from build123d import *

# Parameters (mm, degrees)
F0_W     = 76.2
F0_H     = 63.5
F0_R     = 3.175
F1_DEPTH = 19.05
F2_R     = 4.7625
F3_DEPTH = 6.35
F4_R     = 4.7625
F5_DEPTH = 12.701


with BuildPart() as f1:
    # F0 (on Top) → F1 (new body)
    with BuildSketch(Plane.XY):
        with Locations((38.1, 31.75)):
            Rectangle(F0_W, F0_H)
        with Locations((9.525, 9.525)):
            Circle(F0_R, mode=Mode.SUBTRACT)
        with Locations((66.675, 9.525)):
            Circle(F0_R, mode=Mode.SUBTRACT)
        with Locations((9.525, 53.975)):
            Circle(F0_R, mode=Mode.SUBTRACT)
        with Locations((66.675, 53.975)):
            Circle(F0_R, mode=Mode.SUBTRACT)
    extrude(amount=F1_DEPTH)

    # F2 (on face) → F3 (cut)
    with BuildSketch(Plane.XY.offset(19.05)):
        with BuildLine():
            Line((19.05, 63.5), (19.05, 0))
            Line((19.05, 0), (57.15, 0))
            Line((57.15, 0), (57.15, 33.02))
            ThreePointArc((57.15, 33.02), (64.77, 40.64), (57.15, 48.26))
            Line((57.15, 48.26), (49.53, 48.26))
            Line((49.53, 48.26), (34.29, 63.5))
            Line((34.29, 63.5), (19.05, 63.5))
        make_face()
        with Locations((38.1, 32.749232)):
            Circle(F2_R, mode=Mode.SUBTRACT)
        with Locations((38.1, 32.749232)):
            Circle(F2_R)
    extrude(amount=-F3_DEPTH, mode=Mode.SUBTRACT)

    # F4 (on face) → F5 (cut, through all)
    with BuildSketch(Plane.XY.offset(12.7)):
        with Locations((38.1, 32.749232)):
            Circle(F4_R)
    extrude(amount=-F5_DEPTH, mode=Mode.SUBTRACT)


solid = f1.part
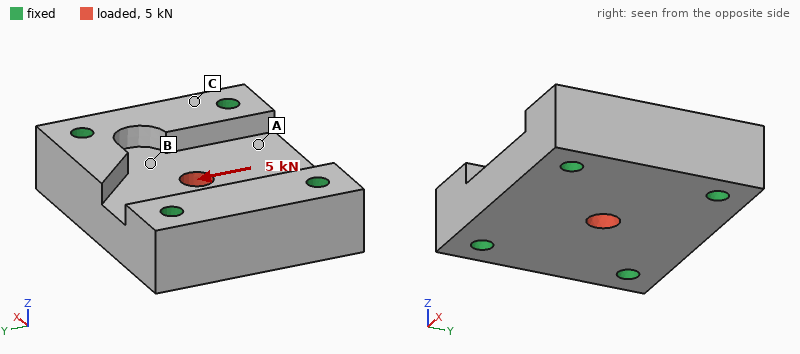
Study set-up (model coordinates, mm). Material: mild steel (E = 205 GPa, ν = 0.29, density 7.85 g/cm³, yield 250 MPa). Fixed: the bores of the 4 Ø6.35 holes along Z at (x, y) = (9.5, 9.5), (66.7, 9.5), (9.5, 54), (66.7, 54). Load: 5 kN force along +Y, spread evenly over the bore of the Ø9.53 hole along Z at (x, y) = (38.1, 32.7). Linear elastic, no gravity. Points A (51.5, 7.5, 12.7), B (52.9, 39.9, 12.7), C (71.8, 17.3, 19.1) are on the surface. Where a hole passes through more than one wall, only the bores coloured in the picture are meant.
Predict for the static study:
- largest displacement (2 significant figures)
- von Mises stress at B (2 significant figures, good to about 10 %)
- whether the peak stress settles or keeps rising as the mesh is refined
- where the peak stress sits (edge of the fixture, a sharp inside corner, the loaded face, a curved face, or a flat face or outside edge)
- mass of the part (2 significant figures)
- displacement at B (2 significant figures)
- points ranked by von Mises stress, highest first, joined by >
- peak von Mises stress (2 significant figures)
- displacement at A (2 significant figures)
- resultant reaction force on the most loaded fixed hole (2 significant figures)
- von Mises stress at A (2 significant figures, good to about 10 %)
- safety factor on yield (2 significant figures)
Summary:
1.5 µm
6.9 MPa
settles
the loaded face
580 g
0.63 µm
B > A > C
23 MPa
0.61 µm
1.5 kN
4.4 MPa
11
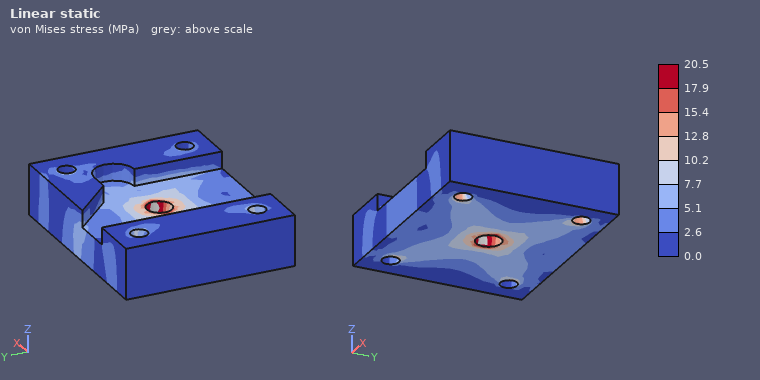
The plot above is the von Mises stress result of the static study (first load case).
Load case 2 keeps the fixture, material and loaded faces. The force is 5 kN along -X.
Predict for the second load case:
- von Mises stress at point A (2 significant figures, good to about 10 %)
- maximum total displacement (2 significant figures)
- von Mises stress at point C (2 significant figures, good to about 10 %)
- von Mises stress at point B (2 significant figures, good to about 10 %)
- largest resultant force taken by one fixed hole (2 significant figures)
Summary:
2.7 MPa
1.2 µm
1.8 MPa
6.9 MPa
1.4 kN
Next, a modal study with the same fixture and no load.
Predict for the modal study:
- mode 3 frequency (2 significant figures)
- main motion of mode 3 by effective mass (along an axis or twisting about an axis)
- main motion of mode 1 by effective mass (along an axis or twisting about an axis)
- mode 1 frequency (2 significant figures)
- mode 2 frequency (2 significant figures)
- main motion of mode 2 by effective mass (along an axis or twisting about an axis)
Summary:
25 kHz
along Y
along Z
17 kHz
21 kHz
twisting about X
